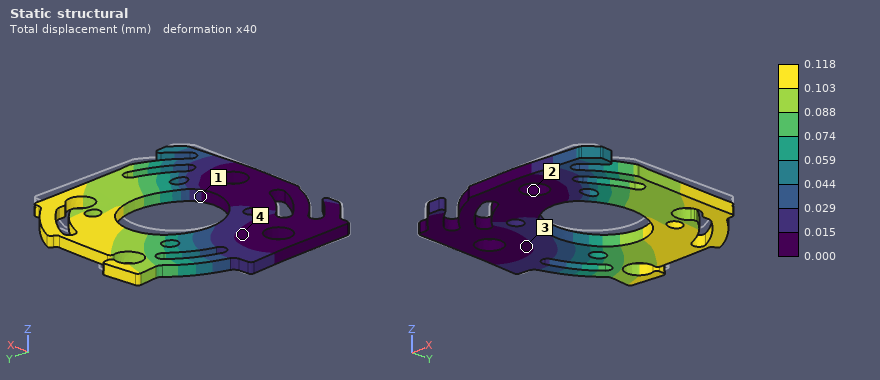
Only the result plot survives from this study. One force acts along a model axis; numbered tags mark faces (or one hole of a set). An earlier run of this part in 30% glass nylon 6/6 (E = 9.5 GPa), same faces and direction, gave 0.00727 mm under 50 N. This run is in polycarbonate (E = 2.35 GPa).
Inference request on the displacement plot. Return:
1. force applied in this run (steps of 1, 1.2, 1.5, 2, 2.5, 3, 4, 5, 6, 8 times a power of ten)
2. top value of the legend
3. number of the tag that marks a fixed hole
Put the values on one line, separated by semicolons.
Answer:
200 N; 0.118 mm; 2
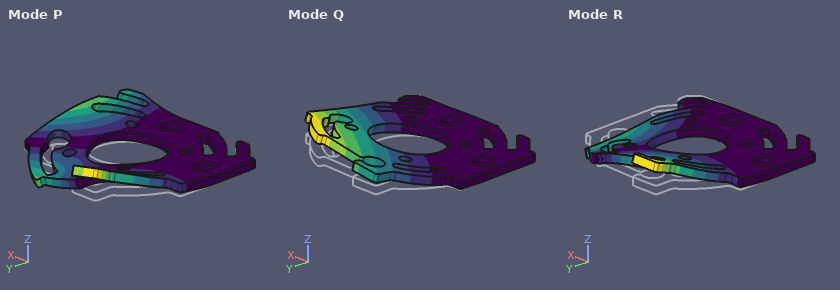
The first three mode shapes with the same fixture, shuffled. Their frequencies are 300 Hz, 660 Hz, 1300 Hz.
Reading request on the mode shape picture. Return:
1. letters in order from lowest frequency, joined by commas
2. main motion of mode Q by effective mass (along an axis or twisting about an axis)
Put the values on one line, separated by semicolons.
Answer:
Q, R, P; along Z
